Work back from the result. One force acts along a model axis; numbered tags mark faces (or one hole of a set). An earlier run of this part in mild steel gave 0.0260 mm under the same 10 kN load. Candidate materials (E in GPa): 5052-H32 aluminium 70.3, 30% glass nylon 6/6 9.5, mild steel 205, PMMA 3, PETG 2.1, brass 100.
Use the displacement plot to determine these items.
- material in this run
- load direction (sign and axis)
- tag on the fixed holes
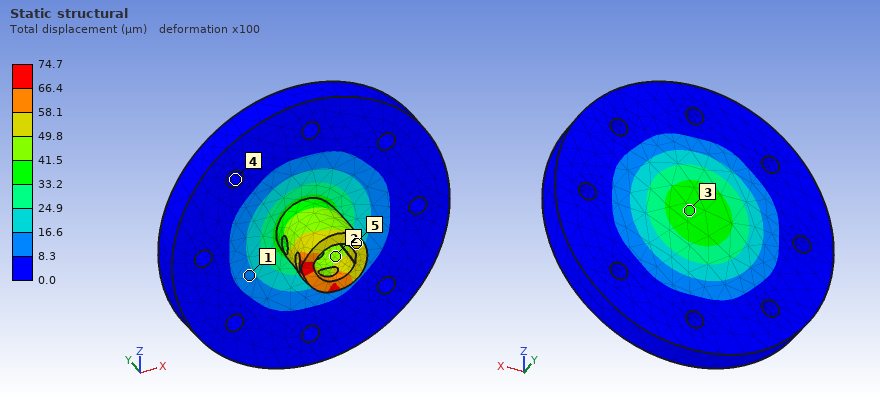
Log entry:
5052-H32 aluminium
+Y
4
